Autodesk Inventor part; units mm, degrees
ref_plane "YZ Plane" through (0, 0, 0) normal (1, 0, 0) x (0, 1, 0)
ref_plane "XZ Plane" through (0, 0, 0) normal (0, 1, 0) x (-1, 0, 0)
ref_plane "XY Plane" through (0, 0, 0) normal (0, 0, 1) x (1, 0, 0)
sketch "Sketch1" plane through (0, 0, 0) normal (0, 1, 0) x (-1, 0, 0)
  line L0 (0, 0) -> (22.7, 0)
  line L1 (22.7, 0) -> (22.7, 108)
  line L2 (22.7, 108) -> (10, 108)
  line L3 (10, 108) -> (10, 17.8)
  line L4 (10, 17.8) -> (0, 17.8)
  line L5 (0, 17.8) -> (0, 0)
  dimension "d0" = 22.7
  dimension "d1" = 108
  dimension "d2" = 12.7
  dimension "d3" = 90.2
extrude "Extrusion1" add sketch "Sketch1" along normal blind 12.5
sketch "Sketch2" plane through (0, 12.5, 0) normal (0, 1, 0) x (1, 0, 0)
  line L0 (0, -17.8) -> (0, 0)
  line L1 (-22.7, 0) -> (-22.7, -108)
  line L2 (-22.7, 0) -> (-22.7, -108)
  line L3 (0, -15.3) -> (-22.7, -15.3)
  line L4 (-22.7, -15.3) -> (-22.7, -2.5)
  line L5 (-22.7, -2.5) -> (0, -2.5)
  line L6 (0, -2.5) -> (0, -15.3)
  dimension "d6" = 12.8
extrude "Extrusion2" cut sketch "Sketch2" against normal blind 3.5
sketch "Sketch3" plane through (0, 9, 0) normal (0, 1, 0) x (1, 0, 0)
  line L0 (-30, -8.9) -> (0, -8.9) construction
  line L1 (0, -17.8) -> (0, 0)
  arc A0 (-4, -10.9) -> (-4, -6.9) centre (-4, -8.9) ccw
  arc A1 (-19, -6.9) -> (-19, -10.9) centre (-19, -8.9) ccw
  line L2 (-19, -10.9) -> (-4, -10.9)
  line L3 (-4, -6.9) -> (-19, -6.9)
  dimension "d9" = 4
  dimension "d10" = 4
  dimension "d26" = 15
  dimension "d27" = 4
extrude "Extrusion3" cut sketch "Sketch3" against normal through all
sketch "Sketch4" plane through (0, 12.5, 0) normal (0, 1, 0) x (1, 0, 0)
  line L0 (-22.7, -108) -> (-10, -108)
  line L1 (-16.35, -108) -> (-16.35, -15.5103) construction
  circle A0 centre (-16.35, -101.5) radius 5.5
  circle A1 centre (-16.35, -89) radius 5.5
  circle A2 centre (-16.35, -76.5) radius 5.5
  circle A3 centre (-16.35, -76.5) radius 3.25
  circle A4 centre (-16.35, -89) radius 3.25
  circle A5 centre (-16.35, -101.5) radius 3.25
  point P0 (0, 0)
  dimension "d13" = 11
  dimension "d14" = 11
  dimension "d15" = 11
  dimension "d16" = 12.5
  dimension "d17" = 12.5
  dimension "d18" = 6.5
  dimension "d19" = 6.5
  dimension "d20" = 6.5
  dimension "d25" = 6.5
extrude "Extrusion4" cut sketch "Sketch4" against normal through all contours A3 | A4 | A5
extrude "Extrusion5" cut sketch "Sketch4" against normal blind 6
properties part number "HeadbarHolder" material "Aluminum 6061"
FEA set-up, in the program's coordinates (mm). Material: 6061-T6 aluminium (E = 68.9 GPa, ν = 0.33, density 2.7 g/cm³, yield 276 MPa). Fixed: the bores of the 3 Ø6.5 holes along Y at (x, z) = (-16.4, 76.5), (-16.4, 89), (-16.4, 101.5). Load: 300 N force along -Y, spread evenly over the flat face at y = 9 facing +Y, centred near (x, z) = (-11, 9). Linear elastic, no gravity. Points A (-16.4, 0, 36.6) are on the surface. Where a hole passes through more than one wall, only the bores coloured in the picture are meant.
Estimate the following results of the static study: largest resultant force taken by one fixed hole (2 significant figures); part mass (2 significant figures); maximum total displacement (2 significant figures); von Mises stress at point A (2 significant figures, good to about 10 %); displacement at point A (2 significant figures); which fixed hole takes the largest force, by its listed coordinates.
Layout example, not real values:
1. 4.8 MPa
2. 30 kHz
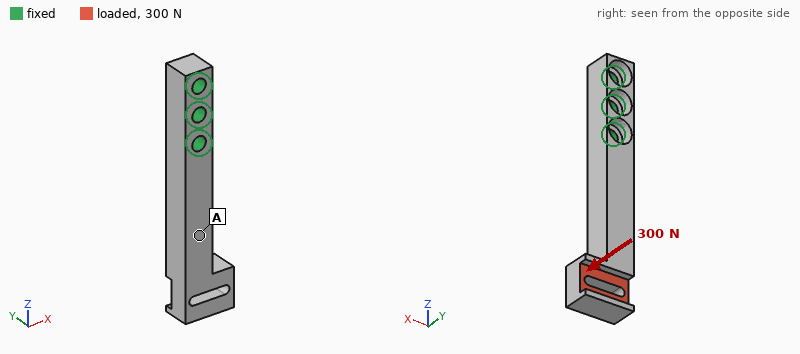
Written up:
1. 900 N
2. 41 g
3. 0.42 mm
4. 26 MPa
5. 0.16 mm
6. (-16.4, 76.5)
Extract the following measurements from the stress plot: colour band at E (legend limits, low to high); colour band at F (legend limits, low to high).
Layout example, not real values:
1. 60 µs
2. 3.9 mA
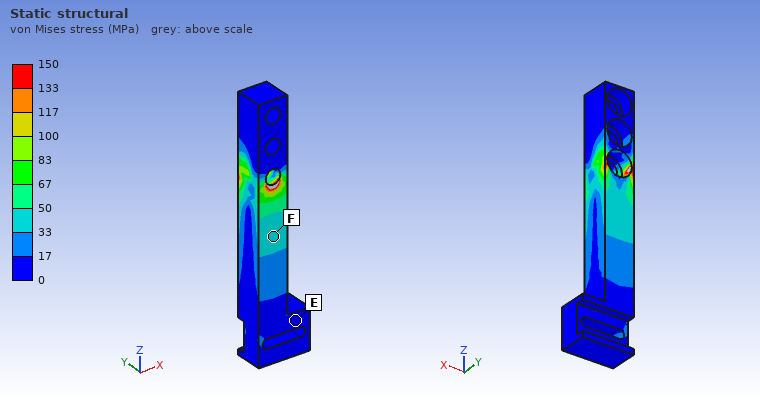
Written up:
1. 0 to 17 MPa
2. 33 to 50 MPa
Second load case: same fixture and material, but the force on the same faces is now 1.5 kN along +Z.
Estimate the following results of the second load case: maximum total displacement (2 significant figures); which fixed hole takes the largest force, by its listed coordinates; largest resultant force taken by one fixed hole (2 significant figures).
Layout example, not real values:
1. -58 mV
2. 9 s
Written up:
1. 0.28 mm
2. (-16.4, 76.5)
3. 1.2 kN
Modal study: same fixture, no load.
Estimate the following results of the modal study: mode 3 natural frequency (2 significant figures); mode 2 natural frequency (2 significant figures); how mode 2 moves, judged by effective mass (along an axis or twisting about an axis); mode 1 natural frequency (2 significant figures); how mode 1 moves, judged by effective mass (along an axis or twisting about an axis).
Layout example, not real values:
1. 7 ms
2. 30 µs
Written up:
1. 6100 Hz
2. 1500 Hz
3. along X
4. 1300 Hz
5. along Y
